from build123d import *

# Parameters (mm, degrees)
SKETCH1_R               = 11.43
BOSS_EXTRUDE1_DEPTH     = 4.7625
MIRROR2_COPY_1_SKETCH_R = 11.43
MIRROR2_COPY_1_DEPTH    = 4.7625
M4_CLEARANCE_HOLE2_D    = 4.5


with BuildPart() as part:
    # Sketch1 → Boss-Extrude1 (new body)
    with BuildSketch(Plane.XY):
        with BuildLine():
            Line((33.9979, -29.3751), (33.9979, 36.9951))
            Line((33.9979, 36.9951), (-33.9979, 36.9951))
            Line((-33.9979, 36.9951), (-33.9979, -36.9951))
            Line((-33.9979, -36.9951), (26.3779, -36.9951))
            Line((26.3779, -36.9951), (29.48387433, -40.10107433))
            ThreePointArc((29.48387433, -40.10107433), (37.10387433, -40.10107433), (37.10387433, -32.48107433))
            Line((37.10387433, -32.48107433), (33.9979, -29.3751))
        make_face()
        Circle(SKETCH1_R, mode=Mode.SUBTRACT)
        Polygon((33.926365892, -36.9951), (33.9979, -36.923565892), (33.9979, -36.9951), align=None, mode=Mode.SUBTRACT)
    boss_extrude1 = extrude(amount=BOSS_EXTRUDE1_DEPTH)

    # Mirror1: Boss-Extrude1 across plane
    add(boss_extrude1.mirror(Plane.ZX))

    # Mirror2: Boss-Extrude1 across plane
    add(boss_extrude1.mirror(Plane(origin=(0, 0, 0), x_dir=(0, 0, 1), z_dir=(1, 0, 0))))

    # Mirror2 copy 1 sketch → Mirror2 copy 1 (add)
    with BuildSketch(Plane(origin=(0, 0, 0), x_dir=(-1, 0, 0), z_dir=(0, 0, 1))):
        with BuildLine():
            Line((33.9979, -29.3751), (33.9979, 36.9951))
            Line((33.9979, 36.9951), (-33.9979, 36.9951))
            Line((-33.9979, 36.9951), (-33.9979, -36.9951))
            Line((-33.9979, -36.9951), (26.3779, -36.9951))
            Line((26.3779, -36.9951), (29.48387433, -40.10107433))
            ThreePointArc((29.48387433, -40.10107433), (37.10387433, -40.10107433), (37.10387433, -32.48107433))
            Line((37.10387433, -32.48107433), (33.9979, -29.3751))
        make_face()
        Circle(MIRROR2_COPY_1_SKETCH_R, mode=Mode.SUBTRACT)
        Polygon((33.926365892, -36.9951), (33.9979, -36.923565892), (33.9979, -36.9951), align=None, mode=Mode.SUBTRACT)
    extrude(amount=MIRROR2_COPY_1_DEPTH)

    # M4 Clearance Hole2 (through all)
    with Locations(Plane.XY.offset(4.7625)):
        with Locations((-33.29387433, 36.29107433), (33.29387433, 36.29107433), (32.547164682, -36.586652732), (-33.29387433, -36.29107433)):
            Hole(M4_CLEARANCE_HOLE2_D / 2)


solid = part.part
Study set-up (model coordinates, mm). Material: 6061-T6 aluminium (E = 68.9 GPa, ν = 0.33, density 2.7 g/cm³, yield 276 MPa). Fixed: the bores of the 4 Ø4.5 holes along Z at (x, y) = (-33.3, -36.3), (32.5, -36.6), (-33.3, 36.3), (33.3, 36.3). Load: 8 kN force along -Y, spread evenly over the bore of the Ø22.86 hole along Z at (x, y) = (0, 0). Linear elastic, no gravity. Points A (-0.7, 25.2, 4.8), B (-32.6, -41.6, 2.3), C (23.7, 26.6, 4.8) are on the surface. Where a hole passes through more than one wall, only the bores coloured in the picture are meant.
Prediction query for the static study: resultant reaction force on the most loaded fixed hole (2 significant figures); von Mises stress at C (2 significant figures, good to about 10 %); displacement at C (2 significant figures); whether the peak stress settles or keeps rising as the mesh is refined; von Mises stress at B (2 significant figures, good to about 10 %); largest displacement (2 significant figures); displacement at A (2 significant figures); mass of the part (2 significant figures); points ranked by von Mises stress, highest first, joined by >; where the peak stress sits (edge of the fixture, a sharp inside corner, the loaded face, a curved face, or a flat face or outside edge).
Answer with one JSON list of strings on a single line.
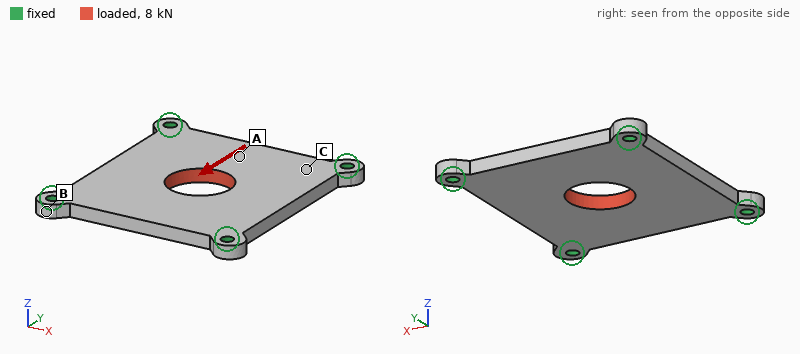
["2.4 kN", "29 MPa", "9.6 µm", "keeps rising", "15 MPa", "22 µm", "19 µm", "62 g", "C > B > A", "edge of the fixture"]
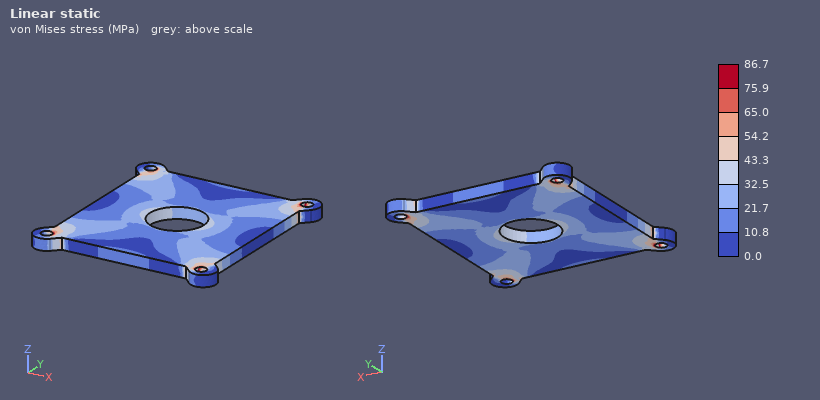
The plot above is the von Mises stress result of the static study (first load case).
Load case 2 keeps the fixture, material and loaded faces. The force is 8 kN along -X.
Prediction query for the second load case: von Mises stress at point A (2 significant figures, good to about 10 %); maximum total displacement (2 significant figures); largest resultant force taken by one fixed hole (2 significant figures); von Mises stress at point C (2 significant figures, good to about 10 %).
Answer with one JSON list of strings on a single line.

["21 MPa", "25 µm", "2.4 kN", "30 MPa"]
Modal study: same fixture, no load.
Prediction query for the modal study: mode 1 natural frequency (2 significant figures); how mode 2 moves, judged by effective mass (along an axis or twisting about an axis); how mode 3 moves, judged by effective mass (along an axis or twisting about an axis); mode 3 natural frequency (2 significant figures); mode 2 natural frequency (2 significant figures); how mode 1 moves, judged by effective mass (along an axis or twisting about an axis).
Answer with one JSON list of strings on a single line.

["3000 Hz", "twisting about Y", "twisting about X", "5700 Hz", "5200 Hz", "along Z"]
